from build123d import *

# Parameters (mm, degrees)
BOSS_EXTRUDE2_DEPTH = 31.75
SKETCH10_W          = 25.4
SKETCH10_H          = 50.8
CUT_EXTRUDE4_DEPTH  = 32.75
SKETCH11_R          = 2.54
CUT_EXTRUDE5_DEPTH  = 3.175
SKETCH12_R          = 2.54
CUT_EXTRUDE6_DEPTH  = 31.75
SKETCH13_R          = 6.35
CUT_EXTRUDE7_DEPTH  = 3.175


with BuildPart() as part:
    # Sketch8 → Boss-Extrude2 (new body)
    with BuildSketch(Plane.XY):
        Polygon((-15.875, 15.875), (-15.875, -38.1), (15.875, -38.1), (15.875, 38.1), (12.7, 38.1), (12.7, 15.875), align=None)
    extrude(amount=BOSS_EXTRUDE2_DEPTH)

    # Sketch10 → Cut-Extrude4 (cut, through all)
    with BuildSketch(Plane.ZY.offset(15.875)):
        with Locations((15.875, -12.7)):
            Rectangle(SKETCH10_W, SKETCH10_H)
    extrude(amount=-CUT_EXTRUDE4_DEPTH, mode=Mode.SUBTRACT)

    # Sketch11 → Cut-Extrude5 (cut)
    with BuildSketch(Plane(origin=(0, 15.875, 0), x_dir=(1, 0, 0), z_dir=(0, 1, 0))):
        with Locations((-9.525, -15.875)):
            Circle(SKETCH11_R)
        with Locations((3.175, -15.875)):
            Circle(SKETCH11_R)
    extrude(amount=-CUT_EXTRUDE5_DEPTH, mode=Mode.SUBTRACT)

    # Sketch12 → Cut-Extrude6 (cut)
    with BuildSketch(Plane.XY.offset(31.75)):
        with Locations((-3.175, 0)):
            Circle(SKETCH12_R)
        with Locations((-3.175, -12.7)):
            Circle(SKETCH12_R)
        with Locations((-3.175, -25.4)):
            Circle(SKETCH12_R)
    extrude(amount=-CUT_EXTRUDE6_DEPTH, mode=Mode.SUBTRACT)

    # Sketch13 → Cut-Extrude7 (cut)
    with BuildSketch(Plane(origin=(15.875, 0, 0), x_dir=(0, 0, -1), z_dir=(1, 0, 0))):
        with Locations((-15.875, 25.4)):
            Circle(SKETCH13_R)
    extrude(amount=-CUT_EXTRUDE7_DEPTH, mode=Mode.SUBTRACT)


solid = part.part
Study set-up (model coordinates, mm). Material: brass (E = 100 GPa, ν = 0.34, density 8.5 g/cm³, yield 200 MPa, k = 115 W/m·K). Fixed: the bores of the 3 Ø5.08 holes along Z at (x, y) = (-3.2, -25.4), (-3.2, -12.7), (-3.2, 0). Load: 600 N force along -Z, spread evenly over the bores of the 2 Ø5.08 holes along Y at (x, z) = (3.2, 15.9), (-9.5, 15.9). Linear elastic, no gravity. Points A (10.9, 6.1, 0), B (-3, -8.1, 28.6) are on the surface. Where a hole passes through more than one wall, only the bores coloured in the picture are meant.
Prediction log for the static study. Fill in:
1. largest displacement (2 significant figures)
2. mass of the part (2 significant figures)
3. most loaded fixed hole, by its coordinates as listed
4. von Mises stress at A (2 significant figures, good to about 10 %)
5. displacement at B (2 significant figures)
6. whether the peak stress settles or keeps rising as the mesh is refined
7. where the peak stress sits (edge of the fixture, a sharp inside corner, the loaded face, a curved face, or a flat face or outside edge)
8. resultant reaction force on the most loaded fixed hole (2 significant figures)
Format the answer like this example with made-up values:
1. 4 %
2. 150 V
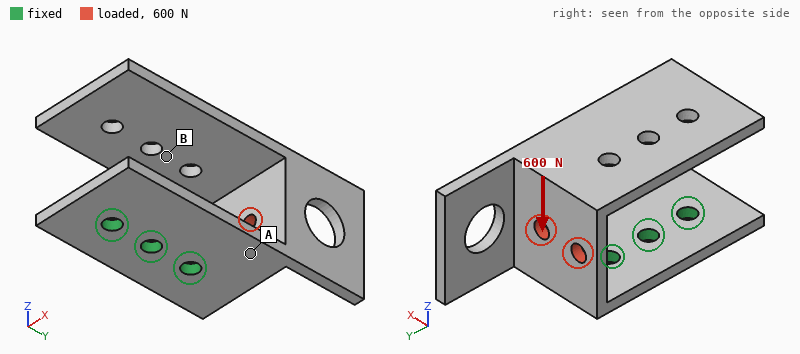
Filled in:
1. 0.34 mm
2. 130 g
3. (-3.2, 0)
4. 55 MPa
5. 0.20 mm
6. keeps rising
7. edge of the fixture
8. 790 N
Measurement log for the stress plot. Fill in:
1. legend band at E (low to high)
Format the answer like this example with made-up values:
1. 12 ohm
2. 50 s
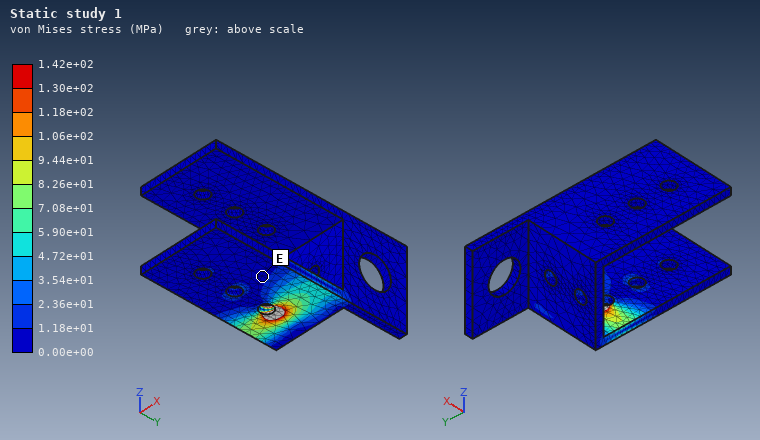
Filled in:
1. 0.00e+00 to 1.18e+01 MPa
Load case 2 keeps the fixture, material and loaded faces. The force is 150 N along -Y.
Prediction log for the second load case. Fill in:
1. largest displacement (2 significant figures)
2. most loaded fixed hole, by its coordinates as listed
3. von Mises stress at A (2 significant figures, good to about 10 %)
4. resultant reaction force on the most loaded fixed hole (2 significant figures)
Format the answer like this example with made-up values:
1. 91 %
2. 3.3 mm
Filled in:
1. 0.23 mm
2. (-3.2, 0)
3. 32 MPa
4. 130 N
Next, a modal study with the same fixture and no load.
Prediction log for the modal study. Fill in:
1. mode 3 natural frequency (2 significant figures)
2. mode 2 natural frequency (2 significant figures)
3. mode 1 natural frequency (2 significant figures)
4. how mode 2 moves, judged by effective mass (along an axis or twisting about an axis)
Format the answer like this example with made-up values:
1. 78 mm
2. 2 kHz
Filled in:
1. 770 Hz
2. 460 Hz
3. 330 Hz
4. along X
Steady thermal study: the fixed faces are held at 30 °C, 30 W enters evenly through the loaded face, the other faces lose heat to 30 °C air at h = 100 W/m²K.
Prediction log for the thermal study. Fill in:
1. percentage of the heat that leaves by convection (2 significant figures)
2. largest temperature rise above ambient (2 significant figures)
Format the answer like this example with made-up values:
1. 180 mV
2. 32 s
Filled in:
1. 56 %
2. 44 K
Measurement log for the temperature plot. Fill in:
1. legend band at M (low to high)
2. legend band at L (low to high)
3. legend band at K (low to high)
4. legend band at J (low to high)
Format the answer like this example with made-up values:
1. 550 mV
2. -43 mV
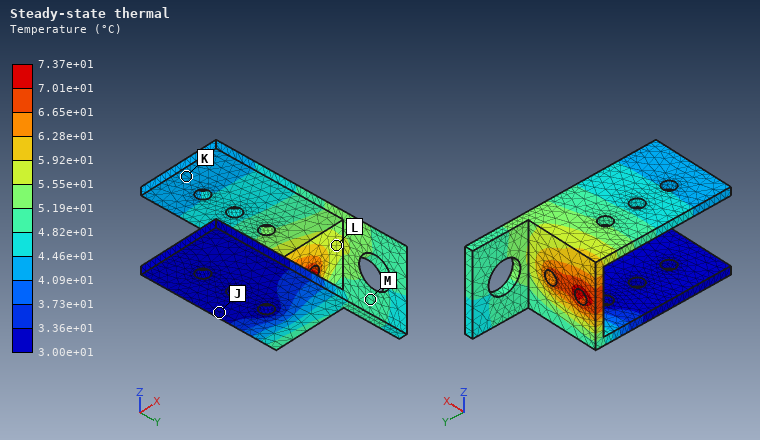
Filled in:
1. 4.82e+01 to 5.19e+01 °C
2. 5.55e+01 to 5.92e+01 °C
3. 4.09e+01 to 4.46e+01 °C
4. 3.00e+01 to 3.36e+01 °C
